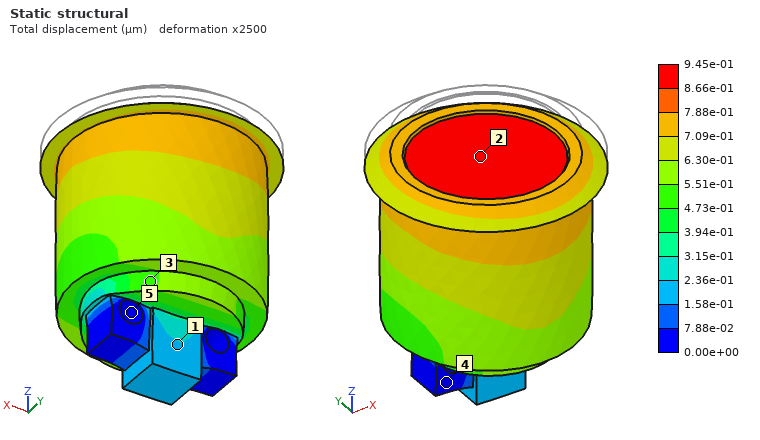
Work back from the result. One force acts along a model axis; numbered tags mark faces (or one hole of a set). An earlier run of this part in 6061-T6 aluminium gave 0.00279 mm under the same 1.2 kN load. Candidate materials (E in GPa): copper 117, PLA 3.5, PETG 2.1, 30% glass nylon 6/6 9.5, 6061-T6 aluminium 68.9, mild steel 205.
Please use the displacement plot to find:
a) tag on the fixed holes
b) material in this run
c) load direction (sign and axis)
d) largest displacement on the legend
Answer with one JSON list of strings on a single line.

["5", "mild steel", "-Z", "9.45e-01 µm"]
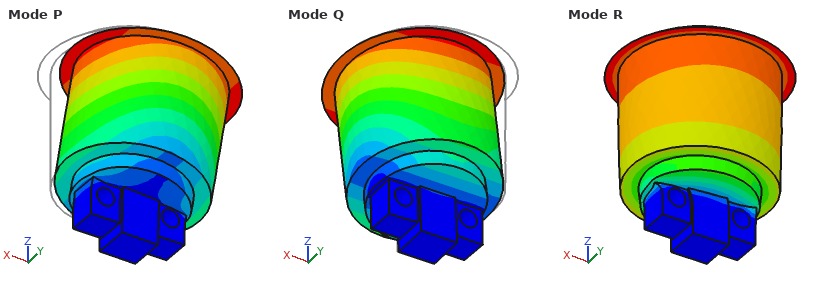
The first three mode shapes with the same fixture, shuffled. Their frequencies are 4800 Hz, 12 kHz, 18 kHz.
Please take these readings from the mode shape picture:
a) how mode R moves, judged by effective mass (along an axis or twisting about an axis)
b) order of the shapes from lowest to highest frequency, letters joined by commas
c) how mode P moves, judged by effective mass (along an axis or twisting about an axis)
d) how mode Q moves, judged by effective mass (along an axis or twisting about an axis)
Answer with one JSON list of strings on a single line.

["twisting about Z", "Q, P, R", "along X", "along Y"]
